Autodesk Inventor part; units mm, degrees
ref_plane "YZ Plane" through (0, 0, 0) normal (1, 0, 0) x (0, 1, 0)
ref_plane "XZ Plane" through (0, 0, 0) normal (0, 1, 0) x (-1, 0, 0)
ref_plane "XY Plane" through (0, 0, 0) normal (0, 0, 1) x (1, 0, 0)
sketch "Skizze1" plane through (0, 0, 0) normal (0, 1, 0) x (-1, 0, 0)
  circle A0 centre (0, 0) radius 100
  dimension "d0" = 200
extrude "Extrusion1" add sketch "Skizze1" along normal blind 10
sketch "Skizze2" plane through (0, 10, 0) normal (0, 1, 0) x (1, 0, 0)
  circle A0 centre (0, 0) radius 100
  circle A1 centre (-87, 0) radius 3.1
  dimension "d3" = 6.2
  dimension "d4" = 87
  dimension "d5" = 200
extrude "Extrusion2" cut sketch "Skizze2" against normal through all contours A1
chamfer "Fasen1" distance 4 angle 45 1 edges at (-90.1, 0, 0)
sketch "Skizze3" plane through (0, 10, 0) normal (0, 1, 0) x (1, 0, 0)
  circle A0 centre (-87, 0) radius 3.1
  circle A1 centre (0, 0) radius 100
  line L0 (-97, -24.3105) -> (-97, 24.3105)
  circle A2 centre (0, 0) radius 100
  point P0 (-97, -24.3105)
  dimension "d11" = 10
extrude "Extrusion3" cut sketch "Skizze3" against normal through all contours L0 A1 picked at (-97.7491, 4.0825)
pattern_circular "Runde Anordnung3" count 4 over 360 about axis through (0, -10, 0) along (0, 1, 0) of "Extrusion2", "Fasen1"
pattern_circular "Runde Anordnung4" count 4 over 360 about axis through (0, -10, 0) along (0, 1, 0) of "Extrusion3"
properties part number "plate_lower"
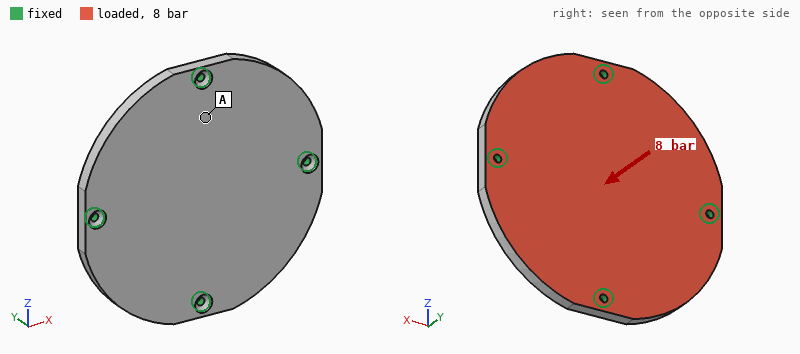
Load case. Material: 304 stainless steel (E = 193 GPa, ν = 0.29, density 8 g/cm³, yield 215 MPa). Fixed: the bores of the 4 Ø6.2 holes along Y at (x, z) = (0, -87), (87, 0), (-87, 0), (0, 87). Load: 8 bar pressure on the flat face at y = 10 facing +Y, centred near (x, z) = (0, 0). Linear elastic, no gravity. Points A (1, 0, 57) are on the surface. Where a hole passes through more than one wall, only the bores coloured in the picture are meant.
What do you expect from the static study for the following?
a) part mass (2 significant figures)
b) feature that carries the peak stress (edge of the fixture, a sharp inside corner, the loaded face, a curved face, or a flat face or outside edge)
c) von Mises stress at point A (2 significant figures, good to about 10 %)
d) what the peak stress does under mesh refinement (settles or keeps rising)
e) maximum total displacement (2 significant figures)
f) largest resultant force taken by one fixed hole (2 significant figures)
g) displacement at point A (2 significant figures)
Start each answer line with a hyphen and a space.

- 2.5 kg
- edge of the fixture
- 32 MPa
- keeps rising
- 0.11 mm
- 7.0 kN
- 0.056 mm
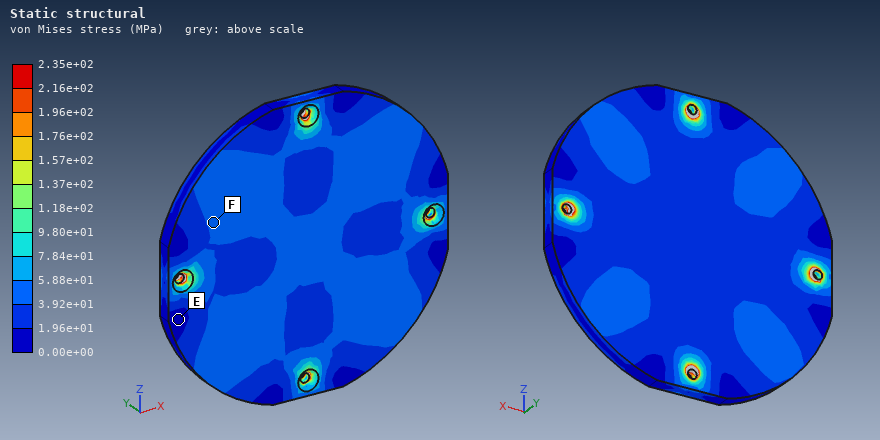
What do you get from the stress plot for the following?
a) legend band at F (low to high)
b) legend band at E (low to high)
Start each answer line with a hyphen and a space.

- 3.92e+01 to 5.88e+01 MPa
- 0.00e+00 to 1.96e+01 MPa
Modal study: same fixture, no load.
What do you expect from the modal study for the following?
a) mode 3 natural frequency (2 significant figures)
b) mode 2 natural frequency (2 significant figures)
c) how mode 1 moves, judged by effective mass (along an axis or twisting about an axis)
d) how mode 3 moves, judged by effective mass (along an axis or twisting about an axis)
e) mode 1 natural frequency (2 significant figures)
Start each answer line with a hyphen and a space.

- 2300 Hz
- 2000 Hz
- along Y
- twisting about Z
- 1900 Hz
